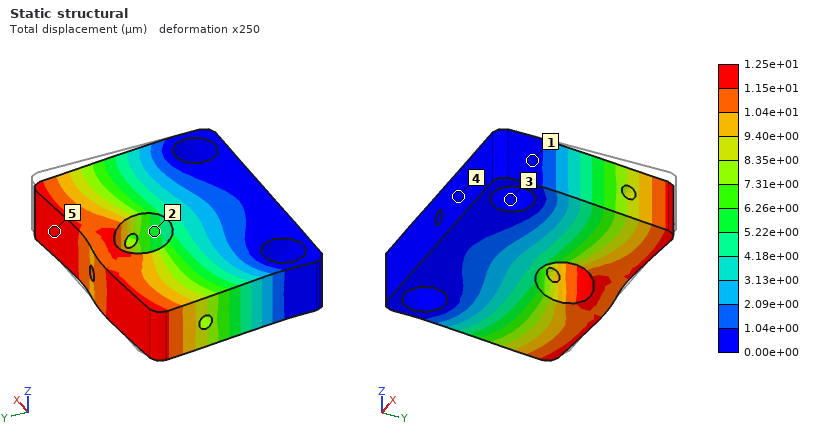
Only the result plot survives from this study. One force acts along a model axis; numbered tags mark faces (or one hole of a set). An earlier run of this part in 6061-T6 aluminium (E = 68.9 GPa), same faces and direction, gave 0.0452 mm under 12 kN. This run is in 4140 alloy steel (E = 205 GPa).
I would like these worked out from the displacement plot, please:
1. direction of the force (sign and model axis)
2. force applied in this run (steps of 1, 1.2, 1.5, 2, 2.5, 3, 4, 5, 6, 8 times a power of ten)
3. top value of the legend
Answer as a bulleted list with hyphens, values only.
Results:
- -X
- 10 kN
- 1.25e+01 µm
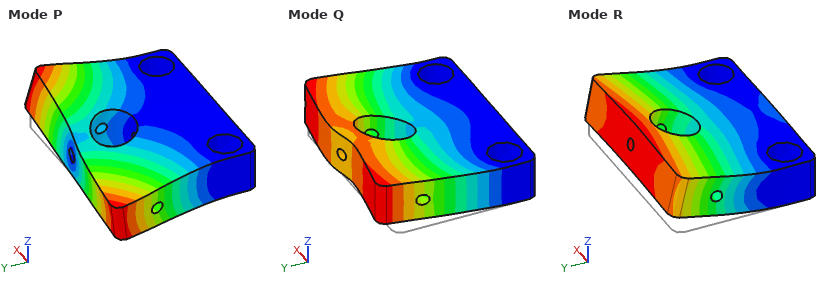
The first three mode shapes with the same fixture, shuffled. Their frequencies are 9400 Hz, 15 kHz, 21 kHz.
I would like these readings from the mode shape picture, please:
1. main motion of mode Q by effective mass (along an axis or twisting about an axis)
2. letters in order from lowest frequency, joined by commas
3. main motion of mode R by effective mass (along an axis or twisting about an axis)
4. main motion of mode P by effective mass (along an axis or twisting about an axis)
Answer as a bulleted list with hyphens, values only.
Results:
- along X
- R, P, Q
- along Z
- twisting about Y
